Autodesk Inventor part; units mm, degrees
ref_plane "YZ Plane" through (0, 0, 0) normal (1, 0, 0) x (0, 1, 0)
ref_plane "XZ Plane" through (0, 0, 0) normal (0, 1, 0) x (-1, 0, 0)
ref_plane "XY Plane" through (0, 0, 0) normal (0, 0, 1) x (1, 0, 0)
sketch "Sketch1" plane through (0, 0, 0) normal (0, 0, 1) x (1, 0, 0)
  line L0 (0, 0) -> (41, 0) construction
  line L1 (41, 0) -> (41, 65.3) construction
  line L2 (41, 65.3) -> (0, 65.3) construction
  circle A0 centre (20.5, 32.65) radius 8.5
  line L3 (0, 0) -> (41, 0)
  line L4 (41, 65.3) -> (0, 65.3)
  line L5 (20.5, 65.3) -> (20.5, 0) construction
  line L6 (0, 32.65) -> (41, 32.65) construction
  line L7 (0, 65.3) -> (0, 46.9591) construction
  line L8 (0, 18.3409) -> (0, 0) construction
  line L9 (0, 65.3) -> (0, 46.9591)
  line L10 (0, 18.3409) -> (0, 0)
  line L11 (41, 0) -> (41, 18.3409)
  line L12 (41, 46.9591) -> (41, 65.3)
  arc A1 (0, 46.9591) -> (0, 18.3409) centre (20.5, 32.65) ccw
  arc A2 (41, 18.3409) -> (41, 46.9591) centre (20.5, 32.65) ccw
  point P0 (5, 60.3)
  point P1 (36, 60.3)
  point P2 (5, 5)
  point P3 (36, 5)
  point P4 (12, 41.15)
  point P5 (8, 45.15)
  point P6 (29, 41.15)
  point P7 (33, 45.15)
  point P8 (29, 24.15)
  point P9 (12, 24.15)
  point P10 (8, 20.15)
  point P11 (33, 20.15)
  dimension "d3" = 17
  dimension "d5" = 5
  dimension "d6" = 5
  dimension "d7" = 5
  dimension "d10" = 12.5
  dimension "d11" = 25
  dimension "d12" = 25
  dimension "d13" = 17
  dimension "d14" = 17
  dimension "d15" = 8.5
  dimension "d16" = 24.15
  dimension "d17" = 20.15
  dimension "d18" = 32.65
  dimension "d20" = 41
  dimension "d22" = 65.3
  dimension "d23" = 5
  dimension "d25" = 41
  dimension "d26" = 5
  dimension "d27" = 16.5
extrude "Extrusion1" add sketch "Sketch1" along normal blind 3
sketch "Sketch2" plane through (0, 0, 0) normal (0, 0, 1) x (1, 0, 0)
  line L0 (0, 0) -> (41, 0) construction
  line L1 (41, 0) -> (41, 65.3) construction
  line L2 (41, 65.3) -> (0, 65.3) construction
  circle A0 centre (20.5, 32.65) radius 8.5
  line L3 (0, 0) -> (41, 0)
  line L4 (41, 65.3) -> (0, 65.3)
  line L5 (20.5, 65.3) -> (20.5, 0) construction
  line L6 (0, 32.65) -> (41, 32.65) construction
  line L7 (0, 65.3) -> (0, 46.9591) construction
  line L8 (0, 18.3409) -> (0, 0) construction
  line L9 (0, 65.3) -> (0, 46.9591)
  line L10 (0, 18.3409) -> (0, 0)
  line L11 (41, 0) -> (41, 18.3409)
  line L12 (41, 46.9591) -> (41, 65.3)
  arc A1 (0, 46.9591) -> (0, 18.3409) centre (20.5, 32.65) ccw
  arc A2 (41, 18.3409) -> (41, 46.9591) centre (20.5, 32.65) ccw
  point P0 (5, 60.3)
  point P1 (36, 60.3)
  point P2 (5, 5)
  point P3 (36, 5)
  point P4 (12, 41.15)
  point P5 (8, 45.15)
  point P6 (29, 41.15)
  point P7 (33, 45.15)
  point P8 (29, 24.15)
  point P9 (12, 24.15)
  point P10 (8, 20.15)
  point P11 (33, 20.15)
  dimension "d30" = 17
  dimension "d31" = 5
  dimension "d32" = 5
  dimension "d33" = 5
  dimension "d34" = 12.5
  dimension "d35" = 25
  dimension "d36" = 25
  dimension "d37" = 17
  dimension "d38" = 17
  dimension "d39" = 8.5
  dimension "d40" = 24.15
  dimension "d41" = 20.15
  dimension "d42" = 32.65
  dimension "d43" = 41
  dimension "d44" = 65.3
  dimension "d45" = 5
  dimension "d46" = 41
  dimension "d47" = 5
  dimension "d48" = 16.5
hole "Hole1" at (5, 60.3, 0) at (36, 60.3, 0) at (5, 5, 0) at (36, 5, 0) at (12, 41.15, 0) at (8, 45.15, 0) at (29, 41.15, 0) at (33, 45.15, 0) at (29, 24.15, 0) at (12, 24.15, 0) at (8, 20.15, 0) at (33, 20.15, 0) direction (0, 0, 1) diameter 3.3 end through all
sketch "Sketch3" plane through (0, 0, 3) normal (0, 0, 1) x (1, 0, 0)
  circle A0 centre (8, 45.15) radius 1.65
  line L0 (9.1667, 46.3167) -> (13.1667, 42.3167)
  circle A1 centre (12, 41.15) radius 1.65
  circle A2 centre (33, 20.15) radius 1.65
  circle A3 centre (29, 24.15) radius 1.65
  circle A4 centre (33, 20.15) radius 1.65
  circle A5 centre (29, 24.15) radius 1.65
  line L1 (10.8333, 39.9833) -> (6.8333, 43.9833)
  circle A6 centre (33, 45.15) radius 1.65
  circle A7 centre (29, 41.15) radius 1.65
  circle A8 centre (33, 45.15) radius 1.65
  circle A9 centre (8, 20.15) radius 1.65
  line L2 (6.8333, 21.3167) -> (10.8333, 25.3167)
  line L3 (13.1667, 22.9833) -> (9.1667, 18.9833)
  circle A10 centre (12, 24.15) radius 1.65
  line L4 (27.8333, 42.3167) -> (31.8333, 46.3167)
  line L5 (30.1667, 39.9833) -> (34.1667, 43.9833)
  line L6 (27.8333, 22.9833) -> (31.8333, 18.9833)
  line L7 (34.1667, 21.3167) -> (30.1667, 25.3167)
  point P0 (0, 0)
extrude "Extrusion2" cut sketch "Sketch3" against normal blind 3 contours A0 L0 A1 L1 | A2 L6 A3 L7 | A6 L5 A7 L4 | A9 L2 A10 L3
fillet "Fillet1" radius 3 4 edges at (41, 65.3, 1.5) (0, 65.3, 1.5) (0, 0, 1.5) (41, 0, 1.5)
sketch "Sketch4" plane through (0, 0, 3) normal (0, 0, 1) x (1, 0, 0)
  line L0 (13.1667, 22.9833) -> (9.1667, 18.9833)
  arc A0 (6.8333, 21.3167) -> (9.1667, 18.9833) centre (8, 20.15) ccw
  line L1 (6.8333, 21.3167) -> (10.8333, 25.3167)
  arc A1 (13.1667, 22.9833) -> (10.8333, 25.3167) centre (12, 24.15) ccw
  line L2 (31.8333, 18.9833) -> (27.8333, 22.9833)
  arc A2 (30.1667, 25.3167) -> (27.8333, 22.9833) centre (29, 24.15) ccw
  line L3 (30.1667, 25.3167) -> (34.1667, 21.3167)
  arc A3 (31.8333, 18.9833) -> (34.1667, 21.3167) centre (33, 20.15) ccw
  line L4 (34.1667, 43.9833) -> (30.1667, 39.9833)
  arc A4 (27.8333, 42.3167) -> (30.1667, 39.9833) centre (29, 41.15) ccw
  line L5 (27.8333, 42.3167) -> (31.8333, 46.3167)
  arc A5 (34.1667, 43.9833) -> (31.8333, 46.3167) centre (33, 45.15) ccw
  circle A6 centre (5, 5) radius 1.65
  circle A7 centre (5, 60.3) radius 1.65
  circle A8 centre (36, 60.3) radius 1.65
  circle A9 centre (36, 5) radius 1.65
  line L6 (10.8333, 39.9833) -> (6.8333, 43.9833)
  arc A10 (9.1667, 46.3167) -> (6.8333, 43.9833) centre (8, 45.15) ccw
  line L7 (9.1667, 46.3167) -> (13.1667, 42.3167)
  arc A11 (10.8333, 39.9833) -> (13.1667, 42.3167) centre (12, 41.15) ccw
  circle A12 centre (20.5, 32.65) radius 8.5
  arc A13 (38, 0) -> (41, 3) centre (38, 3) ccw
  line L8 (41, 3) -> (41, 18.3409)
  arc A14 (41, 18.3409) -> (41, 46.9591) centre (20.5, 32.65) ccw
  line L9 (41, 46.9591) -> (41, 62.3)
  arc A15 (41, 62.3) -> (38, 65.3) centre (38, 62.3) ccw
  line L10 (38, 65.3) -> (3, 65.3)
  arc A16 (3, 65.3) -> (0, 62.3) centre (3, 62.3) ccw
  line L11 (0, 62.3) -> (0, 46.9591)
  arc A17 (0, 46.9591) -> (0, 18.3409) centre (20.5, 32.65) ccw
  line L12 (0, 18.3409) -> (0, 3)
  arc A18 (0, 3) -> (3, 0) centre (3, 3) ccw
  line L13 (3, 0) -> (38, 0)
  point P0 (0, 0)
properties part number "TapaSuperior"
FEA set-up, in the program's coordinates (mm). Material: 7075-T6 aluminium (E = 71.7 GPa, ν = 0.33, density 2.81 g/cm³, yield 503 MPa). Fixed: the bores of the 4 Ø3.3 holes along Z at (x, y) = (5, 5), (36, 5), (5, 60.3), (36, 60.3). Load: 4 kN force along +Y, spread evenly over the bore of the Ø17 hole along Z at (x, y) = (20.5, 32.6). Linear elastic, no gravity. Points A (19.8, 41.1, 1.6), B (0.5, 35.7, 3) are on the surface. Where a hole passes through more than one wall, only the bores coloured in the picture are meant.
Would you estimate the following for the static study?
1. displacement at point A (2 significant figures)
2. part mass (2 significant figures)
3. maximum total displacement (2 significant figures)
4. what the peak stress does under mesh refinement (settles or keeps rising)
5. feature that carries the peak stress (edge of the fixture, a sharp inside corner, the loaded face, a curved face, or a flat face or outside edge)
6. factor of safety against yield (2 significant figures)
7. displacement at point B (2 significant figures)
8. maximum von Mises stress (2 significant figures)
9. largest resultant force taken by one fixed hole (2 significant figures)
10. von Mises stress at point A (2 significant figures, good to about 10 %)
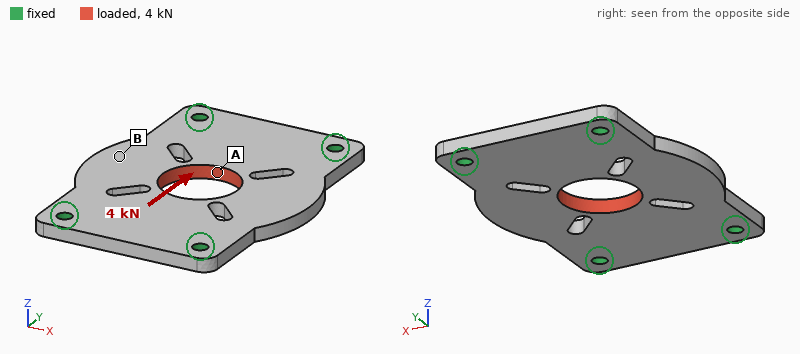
9.6 µm
21 g
13 µm
settles
a curved face
4.5
5.2 µm
110 MPa
1.0 kN
22 MPa
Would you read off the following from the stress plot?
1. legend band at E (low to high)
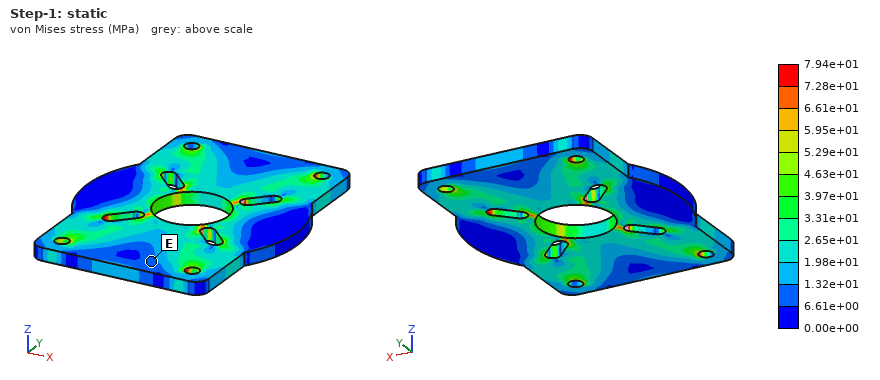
6.61e+00 to 1.32e+01 MPa
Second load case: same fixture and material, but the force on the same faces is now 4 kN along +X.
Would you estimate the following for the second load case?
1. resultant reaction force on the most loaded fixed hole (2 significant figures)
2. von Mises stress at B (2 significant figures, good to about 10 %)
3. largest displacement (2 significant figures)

1.2 kN
22 MPa
23 µm
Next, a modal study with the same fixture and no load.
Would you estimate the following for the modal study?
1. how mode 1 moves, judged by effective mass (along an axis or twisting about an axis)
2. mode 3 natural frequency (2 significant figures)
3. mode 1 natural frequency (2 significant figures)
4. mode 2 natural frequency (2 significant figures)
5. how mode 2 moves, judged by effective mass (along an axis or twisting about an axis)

along Z
8600 Hz
4600 Hz
5600 Hz
twisting about Y
